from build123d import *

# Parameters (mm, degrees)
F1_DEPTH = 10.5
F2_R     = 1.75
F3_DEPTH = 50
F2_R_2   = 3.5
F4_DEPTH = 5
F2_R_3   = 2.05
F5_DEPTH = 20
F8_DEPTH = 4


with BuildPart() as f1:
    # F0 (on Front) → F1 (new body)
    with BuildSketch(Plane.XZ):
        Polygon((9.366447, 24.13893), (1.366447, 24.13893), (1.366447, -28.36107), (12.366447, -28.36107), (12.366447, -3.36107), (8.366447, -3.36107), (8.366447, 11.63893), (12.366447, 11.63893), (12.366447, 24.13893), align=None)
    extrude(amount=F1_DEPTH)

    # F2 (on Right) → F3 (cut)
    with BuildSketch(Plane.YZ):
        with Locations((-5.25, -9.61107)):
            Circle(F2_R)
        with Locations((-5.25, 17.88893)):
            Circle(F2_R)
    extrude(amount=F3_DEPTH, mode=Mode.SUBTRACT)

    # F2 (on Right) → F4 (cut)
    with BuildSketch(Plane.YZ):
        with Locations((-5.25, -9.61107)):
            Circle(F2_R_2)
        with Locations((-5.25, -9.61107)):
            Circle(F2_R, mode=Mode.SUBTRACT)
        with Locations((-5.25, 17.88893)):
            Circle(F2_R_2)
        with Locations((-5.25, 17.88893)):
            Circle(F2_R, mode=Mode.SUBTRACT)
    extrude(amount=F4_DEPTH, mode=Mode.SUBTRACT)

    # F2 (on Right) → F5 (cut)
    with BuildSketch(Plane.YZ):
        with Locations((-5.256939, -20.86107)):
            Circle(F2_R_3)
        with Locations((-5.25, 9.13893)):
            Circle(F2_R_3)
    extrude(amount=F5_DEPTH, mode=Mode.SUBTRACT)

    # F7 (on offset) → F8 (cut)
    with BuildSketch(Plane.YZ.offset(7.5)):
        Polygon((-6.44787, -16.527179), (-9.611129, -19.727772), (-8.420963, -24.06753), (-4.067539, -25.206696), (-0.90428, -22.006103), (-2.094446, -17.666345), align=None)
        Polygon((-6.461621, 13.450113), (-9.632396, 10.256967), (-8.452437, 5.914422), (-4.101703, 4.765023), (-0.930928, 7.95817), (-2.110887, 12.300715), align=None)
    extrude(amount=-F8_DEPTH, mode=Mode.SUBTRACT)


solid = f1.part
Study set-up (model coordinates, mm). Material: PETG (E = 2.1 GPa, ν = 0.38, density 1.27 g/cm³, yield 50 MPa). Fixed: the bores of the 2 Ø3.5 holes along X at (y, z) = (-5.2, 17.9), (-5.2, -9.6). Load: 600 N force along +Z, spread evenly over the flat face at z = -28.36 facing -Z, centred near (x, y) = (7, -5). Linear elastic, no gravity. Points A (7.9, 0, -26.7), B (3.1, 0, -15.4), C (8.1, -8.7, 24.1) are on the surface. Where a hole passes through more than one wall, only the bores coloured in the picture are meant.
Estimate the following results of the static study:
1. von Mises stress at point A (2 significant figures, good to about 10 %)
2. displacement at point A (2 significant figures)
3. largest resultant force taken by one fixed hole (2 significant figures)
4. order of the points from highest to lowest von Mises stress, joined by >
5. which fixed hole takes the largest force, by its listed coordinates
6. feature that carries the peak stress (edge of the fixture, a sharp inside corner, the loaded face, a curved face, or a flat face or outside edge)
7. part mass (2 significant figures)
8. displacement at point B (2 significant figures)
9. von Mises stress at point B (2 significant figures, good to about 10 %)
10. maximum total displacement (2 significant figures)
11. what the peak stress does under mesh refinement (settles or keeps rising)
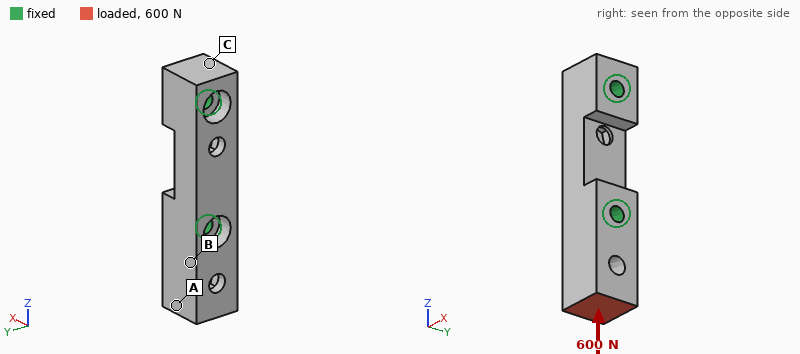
6.4 MPa
0.096 mm
560 N
B > A > C
(-5.2, -9.6)
edge of the fixture
5.7 g
0.051 mm
10 MPa
0.14 mm
keeps rising
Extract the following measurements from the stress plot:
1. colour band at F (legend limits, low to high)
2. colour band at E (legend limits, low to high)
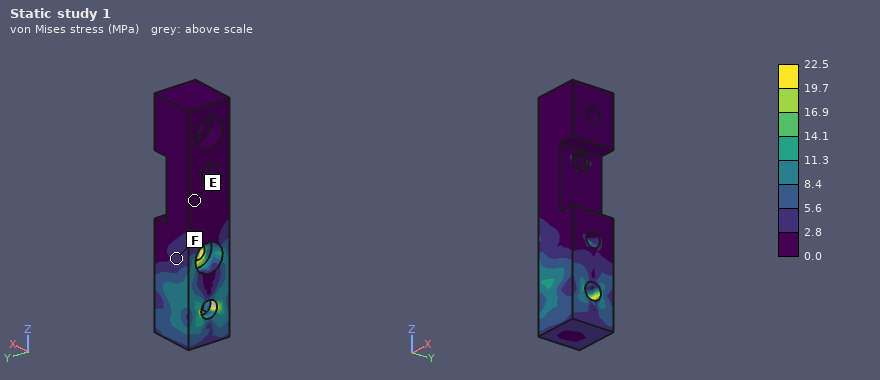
2.8 to 5.6 MPa
0.0 to 2.8 MPa
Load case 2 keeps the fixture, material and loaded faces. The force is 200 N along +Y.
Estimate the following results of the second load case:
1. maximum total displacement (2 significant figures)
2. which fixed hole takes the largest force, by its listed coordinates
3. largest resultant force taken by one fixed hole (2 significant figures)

0.51 mm
(-5.2, -9.6)
250 N
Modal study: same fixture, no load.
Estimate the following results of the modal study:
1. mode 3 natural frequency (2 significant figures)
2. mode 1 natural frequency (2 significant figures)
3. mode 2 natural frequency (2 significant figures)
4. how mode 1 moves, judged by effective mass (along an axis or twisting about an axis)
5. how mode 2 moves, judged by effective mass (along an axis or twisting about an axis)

7700 Hz
3800 Hz
4100 Hz
along Y
along X
